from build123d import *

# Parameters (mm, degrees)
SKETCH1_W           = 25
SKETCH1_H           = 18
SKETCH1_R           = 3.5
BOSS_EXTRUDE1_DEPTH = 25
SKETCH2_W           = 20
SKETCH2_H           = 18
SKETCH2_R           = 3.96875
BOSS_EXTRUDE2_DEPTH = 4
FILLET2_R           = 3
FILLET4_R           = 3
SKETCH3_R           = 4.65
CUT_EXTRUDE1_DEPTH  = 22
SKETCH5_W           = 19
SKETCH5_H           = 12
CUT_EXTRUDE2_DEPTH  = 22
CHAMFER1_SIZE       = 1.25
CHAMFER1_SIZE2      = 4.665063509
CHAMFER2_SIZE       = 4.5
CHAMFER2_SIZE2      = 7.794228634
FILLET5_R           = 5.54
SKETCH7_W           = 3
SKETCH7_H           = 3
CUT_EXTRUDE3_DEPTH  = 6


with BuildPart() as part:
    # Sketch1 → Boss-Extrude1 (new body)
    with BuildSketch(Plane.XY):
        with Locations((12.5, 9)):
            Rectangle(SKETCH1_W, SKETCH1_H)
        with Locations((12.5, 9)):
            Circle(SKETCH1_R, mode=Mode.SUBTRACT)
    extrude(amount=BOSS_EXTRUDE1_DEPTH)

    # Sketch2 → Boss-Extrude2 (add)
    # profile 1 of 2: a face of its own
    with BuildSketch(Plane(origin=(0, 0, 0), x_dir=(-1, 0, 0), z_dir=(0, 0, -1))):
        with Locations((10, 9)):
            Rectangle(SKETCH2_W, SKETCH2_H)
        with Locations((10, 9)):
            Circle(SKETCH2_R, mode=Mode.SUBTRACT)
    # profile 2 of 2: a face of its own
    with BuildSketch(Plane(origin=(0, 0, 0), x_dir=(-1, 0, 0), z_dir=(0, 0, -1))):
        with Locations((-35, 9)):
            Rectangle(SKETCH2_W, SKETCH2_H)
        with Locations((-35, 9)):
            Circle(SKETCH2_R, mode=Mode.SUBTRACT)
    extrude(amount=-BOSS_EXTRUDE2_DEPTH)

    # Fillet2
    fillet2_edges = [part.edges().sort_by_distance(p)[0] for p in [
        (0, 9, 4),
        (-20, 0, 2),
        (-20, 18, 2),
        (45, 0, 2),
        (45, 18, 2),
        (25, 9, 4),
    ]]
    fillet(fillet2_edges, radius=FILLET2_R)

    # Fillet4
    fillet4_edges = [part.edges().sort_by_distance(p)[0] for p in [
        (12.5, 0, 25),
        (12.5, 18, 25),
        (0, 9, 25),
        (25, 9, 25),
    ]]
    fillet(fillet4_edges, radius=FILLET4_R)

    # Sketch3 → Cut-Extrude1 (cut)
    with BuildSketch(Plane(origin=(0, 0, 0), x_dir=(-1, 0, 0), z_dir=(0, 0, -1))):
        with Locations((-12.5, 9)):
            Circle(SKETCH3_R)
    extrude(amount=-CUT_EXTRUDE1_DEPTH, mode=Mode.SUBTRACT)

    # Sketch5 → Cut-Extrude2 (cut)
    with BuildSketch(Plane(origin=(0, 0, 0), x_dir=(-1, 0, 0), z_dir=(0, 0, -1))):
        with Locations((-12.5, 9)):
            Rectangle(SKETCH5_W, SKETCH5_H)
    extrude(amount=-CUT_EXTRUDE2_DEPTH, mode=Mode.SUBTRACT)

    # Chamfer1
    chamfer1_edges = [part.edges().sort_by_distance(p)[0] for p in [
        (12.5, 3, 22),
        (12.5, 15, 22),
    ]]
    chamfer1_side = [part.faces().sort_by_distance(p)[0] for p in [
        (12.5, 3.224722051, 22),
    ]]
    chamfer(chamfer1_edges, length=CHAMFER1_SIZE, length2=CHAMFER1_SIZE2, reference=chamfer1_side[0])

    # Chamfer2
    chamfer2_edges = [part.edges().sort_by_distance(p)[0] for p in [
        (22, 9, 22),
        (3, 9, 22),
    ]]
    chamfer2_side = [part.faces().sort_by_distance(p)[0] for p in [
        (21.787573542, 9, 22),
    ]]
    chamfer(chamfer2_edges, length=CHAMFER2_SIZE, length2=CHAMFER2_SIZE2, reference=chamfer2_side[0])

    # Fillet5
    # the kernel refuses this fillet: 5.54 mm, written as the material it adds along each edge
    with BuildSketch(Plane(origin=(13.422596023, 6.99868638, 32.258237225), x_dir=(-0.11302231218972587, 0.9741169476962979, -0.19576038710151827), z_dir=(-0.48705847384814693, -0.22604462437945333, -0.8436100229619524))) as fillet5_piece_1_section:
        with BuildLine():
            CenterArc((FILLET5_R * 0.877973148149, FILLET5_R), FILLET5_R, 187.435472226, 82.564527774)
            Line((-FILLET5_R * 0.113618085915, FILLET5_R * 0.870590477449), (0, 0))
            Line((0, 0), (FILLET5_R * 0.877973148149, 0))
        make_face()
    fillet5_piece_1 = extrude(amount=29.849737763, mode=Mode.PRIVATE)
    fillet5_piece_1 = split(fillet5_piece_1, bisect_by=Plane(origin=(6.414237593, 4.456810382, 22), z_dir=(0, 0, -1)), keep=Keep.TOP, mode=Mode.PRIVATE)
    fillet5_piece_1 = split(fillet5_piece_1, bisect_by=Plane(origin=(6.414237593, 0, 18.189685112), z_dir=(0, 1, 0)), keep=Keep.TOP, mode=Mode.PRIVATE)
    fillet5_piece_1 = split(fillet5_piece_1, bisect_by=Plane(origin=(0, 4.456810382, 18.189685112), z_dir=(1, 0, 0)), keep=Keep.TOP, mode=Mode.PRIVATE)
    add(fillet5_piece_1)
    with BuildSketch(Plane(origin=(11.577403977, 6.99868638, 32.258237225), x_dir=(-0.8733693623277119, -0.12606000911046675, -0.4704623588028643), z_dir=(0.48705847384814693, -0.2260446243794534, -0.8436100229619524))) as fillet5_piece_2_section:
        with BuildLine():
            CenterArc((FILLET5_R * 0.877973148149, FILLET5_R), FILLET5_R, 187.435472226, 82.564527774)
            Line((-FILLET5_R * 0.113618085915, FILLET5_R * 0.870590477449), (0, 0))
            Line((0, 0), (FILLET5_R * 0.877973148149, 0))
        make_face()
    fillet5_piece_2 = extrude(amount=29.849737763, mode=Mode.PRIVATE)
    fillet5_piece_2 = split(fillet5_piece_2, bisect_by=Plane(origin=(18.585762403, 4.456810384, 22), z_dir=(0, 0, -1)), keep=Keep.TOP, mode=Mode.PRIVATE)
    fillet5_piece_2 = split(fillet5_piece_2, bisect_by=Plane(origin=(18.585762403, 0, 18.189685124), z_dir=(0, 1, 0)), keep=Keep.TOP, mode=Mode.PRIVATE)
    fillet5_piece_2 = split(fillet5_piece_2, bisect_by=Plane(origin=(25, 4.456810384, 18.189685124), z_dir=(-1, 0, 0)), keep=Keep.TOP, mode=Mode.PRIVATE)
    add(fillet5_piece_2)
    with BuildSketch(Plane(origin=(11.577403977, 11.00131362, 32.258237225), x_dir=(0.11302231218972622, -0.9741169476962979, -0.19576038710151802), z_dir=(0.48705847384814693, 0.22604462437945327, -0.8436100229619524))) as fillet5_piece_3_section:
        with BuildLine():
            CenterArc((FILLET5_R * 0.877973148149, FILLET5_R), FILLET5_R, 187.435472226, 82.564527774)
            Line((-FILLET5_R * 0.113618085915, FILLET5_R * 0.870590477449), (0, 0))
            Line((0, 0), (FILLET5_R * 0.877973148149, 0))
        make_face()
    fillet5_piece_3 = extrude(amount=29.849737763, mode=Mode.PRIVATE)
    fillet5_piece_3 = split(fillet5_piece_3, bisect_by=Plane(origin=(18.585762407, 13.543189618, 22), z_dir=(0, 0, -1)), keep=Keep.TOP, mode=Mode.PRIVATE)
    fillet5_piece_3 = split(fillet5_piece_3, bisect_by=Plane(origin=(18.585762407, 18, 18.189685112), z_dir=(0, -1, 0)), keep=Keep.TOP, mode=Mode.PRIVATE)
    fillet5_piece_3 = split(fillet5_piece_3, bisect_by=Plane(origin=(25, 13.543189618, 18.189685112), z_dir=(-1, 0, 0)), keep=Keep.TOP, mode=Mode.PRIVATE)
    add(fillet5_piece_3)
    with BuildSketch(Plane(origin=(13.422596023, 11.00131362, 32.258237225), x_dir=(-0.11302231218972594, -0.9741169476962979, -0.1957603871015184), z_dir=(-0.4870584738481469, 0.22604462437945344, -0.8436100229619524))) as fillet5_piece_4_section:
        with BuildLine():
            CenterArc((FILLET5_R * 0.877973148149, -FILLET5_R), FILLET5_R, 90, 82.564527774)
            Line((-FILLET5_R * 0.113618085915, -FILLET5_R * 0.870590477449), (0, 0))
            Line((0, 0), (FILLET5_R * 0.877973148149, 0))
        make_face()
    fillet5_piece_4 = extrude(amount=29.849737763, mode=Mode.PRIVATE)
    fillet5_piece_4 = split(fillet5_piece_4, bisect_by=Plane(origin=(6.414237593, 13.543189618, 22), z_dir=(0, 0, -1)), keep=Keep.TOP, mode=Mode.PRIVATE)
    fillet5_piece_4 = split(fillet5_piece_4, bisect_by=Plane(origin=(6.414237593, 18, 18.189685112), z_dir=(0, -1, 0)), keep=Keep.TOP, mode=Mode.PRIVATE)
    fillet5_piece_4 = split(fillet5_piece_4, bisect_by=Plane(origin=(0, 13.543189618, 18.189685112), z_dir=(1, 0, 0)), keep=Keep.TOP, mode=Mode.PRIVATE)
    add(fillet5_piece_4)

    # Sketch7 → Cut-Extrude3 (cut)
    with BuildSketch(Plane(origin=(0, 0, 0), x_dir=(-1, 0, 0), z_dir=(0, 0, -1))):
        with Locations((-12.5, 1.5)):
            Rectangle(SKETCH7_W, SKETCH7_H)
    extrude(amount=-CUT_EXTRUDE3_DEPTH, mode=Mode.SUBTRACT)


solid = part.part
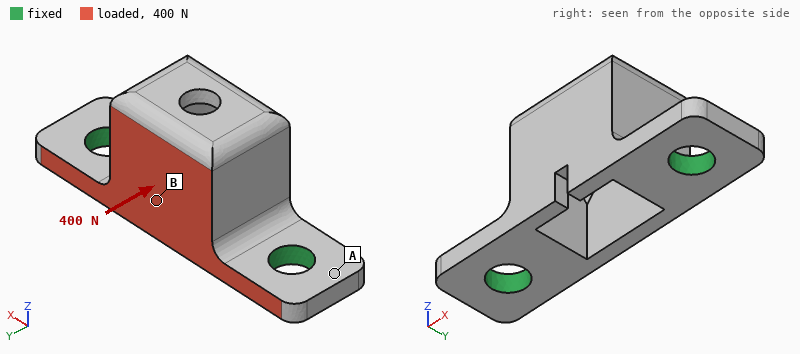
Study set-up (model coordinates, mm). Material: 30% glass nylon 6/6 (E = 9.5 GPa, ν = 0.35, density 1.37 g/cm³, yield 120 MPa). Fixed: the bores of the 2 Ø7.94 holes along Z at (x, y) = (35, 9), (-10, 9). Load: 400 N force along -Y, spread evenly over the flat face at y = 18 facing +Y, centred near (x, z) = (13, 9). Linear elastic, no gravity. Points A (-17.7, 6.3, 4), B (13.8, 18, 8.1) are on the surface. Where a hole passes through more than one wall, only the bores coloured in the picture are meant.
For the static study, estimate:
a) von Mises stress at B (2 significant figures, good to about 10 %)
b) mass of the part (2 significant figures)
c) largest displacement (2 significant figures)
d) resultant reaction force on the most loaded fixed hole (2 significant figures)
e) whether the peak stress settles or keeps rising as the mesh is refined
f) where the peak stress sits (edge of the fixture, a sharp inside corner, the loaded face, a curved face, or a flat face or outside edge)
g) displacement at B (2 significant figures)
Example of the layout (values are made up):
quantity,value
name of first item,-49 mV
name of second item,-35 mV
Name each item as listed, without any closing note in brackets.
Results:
quantity,value
von Mises stress at B,5.8 MPa
mass of the part,12 g
largest displacement,0.15 mm
resultant reaction force on the most loaded fixed hole,210 N
whether the peak stress settles or keeps rising as the mesh is refined,keeps rising
where the peak stress sits,edge of the fixture
displacement at B,0.082 mm
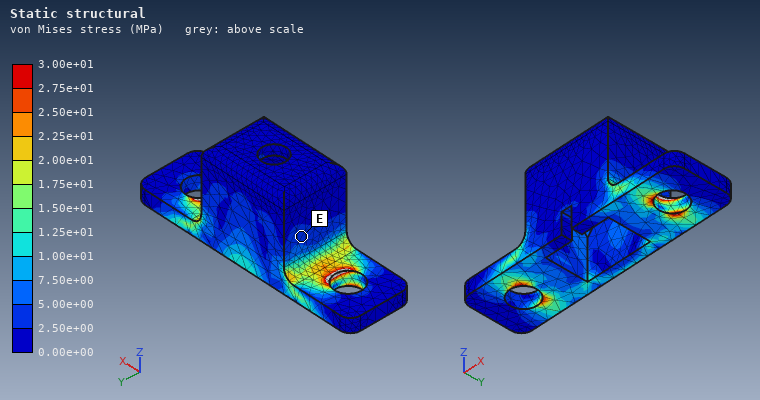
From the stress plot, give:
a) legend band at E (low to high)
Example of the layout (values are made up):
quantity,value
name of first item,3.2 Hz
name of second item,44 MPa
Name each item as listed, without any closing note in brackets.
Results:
quantity,value
legend band at E,2.50e+00 to 5.00e+00 MPa
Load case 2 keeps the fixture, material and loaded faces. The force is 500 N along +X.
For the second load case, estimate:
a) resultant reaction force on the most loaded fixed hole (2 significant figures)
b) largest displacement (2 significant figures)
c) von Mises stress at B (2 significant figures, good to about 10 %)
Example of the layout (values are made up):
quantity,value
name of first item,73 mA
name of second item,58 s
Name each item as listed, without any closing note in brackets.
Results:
quantity,value
resultant reaction force on the most loaded fixed hole,280 N
largest displacement,30 µm
von Mises stress at B,5.7 MPa
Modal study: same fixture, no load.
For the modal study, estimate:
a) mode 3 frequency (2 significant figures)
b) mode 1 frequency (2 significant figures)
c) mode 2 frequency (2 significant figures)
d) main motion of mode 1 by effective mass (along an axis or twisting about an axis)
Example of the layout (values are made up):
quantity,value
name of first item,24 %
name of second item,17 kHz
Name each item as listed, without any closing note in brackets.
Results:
quantity,value
mode 3 frequency,6600 Hz
mode 1 frequency,2400 Hz
mode 2 frequency,6400 Hz
main motion of mode 1 by effective mass,along Y
